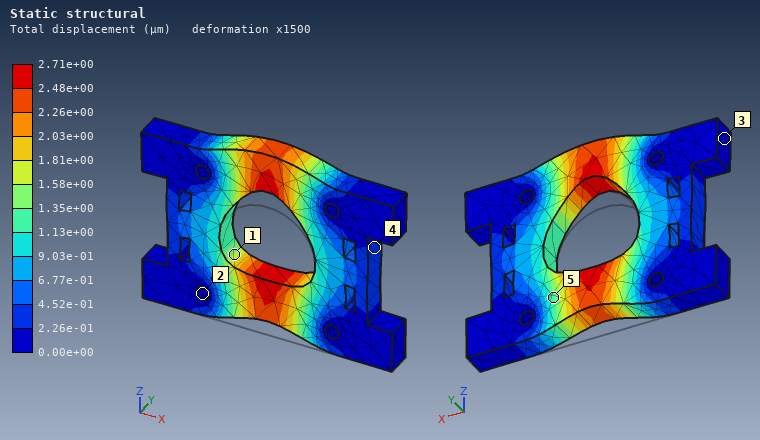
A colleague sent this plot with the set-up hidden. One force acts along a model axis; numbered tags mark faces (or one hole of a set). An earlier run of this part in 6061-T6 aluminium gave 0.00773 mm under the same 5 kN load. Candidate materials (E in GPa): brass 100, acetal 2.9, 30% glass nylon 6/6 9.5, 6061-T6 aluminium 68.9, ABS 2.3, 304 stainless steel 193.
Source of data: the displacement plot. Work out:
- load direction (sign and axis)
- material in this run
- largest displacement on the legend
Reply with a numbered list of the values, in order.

1. +Z
2. 304 stainless steel
3. 2.71e+00 µm
